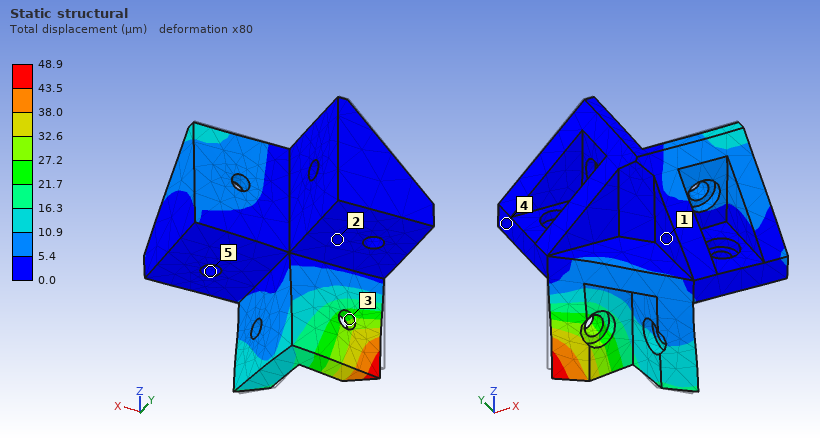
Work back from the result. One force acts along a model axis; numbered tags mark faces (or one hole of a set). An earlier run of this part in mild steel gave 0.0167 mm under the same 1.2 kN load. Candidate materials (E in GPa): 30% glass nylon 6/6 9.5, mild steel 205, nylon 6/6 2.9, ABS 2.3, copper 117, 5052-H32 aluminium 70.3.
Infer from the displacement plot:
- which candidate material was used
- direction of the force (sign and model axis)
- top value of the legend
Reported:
5052-H32 aluminium
-Y
48.9 µm
